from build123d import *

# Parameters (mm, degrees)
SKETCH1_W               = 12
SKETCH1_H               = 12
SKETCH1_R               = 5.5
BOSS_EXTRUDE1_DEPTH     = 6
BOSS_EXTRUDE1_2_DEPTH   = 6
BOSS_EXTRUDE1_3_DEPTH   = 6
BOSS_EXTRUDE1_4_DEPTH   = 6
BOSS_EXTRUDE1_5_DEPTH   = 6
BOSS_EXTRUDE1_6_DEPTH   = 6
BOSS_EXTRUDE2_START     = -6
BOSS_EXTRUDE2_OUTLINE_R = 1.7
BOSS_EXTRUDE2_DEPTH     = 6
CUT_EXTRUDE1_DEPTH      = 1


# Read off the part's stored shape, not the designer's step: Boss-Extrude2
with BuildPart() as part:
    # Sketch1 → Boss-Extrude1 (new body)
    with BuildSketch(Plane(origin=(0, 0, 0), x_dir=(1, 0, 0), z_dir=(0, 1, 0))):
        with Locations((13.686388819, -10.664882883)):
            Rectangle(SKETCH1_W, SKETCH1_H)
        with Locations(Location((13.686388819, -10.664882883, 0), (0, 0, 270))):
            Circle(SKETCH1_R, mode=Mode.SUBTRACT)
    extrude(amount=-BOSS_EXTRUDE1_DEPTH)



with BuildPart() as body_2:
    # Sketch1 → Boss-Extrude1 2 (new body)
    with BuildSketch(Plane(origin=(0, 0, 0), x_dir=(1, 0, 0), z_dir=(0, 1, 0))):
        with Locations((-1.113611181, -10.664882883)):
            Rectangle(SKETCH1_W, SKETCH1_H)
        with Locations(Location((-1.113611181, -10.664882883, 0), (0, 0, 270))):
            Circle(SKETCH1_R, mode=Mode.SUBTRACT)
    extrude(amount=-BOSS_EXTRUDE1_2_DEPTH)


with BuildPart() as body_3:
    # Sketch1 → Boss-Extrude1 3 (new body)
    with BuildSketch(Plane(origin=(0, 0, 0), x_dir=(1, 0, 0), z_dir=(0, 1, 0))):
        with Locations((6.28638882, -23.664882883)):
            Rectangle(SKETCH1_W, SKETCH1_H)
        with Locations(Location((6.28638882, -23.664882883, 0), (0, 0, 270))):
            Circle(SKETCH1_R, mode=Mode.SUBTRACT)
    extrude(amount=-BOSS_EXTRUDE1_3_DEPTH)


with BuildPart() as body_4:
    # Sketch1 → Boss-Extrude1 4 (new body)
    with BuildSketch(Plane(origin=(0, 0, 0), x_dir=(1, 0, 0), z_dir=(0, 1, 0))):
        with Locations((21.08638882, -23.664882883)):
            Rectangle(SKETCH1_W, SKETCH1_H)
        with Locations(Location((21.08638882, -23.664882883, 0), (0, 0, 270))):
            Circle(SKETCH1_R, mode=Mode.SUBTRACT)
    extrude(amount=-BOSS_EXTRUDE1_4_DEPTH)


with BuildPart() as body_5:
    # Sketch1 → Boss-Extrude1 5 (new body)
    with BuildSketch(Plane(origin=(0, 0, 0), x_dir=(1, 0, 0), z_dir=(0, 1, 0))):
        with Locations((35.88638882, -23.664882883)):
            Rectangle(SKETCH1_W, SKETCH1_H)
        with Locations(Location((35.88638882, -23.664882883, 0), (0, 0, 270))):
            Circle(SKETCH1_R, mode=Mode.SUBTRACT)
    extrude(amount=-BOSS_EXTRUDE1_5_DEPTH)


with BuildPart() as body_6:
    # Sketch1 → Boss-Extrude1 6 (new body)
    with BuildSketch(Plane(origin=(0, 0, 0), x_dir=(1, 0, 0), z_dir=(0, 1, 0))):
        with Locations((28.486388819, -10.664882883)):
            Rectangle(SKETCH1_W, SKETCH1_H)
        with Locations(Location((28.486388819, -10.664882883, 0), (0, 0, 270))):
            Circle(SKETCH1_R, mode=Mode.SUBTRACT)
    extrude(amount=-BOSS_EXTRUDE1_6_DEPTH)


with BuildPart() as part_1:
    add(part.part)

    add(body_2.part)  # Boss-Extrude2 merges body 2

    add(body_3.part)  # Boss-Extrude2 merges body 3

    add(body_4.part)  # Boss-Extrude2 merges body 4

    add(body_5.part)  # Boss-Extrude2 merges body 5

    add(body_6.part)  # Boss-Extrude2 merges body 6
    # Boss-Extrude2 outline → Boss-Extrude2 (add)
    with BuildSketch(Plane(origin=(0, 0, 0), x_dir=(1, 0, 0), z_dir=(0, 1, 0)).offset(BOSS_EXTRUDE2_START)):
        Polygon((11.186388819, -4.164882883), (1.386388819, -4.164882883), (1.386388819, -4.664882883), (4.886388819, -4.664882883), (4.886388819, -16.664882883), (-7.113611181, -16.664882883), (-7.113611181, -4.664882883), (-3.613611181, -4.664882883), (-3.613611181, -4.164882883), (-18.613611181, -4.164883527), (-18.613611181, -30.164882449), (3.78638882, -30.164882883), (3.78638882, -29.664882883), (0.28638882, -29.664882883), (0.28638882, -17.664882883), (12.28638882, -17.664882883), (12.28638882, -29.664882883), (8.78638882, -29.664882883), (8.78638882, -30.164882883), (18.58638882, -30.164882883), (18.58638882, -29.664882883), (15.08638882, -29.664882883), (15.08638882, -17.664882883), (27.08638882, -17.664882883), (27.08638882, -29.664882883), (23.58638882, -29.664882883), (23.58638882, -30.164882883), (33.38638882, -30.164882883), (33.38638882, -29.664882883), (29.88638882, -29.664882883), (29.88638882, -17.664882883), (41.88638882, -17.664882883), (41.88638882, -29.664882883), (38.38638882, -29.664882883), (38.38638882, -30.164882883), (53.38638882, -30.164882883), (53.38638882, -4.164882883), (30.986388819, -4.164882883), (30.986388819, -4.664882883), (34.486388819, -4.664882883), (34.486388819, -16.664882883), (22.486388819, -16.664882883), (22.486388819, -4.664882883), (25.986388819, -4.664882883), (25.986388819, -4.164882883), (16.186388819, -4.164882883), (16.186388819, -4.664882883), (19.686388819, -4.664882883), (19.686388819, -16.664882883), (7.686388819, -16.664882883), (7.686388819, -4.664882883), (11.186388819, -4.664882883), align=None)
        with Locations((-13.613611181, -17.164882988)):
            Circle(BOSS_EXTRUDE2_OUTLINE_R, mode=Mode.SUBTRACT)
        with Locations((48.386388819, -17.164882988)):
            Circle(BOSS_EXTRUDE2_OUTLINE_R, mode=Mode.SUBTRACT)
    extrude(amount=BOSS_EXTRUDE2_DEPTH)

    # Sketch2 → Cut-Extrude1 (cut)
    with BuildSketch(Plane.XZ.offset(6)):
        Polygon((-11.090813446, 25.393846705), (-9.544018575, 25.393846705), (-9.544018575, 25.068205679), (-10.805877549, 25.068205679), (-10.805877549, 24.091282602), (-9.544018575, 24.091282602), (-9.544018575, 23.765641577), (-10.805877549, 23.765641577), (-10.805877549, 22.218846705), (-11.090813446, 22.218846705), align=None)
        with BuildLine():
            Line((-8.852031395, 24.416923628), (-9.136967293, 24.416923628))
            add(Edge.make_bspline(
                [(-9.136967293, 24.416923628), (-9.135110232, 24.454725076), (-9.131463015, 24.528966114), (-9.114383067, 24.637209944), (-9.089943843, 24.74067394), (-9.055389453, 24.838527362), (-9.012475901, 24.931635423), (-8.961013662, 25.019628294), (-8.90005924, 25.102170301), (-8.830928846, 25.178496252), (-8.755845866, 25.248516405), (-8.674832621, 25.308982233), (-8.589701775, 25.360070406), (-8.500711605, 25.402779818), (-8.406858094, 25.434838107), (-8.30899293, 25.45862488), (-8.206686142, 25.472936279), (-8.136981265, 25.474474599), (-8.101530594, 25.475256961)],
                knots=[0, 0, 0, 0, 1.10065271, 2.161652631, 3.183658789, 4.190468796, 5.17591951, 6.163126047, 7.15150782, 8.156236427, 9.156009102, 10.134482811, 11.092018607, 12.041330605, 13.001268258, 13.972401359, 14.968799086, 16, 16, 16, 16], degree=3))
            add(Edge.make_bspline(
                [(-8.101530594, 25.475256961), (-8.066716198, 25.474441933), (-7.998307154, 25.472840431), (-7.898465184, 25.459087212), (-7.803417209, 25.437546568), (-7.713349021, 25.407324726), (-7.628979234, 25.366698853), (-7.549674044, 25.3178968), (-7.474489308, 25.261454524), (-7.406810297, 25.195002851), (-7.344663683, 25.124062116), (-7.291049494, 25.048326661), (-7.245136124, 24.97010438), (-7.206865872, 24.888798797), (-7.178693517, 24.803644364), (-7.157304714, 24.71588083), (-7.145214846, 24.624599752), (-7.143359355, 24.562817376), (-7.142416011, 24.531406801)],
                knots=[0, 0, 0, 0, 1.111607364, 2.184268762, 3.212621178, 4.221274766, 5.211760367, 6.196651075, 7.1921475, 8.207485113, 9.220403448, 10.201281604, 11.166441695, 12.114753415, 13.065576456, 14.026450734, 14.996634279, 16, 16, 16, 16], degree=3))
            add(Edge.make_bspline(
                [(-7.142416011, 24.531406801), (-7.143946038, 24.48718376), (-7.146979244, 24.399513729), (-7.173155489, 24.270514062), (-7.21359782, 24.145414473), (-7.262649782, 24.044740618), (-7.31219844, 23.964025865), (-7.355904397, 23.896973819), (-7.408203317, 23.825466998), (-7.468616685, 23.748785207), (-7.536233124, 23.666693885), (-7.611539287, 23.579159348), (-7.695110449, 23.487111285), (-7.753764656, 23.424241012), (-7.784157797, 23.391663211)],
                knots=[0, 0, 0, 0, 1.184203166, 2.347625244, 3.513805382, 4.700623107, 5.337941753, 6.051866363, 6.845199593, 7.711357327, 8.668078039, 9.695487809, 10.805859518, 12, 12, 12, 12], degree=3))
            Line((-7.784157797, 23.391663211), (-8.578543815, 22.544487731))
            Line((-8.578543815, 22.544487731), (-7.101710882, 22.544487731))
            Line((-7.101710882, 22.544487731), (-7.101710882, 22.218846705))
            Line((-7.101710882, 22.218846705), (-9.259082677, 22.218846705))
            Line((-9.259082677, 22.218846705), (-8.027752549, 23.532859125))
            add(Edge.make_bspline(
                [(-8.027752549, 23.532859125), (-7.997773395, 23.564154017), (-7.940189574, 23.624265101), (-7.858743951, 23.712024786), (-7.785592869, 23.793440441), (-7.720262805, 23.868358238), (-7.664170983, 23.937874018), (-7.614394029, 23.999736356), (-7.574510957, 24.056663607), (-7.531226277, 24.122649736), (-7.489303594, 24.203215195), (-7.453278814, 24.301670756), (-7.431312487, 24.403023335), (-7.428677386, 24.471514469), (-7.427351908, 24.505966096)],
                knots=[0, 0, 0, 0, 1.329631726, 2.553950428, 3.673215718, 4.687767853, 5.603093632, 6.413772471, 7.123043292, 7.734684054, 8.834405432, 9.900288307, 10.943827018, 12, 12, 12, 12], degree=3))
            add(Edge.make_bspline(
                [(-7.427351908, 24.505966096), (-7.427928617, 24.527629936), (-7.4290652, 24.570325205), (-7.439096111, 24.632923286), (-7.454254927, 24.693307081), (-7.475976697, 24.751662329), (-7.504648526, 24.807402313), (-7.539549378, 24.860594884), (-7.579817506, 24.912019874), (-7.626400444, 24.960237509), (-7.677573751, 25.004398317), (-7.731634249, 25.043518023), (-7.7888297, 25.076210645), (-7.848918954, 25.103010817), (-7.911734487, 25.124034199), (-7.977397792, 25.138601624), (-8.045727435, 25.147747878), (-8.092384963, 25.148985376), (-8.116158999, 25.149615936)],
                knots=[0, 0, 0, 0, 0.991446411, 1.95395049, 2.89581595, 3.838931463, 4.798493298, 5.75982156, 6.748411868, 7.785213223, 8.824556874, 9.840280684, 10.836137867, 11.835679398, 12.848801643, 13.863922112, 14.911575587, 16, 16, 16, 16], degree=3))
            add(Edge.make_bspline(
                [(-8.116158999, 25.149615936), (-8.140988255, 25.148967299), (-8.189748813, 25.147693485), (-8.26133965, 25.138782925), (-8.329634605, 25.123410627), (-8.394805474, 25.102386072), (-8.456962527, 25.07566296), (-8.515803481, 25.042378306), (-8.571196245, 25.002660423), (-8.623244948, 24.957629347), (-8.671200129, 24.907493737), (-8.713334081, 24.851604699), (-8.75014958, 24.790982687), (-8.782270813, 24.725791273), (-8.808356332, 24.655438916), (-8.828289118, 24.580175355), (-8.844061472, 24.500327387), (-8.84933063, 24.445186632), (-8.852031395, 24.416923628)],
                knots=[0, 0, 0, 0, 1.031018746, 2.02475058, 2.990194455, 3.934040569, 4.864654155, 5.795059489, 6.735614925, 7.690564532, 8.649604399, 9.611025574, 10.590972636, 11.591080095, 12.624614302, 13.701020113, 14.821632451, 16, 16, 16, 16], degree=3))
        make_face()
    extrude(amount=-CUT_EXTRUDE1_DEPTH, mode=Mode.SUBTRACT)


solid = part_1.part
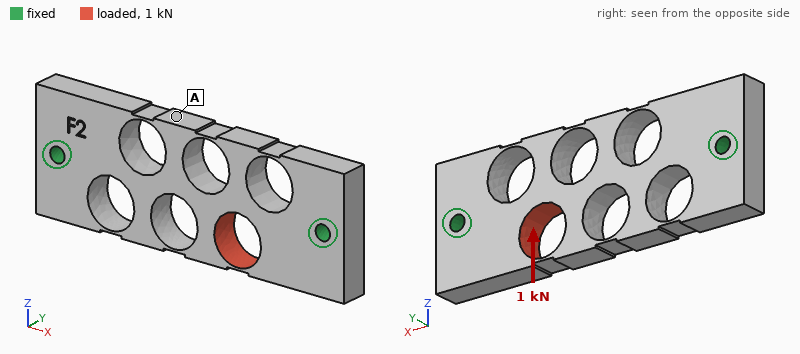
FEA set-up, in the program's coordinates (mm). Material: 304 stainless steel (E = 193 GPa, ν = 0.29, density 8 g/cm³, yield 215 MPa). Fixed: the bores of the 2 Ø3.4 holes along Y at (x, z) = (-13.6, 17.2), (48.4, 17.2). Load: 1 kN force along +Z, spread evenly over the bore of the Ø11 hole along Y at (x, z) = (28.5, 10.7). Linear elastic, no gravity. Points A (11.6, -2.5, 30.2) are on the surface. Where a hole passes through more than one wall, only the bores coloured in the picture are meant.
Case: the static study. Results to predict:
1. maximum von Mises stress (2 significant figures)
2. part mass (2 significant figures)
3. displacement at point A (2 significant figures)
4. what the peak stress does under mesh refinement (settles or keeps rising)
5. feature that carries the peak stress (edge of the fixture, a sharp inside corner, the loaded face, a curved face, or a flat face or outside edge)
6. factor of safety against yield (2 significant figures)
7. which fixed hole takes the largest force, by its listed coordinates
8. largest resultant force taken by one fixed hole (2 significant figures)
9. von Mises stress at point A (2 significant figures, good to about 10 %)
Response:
140 MPa
61 g
10 µm
settles
a flat face or outside edge
1.5
(48.4, 17.2)
720 N
23 MPa
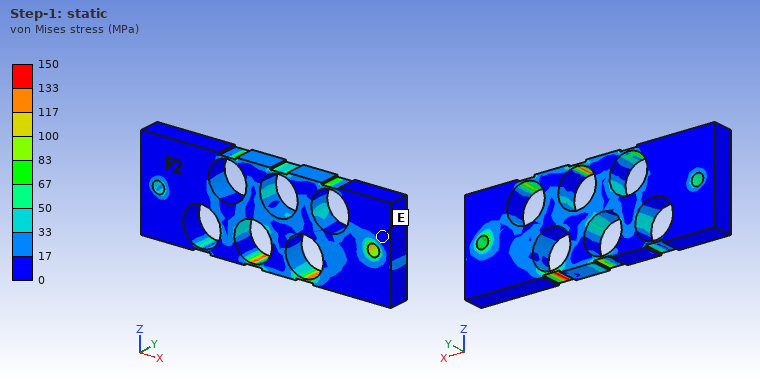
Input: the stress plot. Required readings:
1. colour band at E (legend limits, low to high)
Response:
0 to 17 MPa
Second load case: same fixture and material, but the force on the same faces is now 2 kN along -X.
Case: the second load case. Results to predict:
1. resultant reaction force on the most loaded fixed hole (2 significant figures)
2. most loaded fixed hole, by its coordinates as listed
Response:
1.5 kN
(48.4, 17.2)
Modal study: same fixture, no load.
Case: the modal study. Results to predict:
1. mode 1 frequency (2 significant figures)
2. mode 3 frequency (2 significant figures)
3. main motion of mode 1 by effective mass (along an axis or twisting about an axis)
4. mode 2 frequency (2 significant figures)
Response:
6700 Hz
9600 Hz
along Y
9400 Hz
